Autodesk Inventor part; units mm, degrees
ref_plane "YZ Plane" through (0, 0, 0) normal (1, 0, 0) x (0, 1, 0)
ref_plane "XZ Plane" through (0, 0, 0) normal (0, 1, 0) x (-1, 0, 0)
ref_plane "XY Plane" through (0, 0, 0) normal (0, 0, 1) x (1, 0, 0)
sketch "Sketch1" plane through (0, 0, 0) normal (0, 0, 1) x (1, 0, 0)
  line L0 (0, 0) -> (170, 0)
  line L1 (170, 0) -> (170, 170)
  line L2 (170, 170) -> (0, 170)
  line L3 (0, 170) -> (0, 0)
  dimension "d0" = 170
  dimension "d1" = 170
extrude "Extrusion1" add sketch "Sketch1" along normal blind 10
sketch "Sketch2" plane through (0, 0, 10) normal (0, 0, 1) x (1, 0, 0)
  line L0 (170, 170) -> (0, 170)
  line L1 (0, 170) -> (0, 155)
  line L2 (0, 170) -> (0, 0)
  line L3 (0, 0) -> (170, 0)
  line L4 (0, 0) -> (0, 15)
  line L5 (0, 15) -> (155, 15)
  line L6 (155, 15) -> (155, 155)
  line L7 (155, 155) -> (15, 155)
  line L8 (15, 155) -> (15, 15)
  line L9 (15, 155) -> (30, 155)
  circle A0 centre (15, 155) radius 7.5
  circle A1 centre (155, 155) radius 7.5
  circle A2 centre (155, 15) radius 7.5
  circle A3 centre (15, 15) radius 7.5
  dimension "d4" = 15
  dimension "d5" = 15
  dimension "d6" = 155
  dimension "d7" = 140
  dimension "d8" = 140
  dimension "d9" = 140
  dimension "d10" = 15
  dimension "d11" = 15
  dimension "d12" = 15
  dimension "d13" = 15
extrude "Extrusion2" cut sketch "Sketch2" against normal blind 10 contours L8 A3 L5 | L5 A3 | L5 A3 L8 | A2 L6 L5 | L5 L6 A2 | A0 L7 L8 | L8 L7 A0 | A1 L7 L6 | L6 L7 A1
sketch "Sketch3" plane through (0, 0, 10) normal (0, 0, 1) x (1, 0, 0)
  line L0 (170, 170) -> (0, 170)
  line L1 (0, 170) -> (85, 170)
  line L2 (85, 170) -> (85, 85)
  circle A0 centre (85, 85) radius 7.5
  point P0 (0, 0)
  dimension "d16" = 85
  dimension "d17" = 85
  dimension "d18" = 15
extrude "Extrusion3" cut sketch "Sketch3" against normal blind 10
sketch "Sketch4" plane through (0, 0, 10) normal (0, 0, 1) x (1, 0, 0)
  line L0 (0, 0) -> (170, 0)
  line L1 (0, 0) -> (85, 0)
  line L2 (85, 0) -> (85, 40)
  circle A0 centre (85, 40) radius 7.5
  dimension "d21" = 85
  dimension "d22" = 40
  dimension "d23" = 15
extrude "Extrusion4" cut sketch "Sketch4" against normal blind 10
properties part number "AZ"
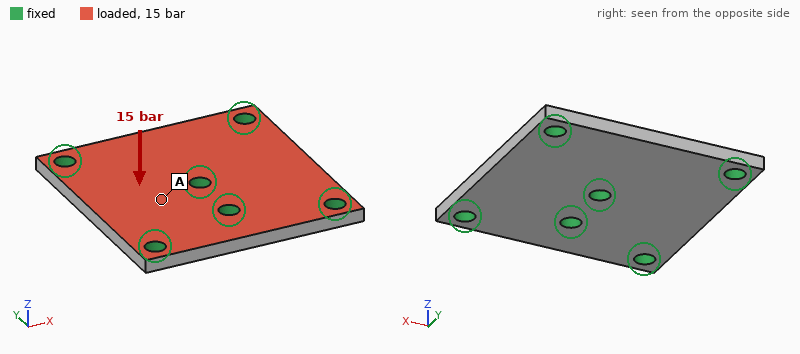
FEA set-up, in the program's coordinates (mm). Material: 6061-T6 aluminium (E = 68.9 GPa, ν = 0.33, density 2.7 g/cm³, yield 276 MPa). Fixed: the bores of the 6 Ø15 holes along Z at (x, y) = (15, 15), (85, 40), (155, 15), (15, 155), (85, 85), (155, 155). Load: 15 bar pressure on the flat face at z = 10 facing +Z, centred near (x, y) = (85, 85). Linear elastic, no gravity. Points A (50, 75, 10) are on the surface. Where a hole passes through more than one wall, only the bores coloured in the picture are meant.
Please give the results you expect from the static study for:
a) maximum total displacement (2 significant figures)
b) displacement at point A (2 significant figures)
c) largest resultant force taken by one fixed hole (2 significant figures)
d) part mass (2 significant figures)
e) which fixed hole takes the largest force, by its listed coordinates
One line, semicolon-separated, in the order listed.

0.18 mm; 0.065 mm; 11 kN; 750 g; (85, 85)
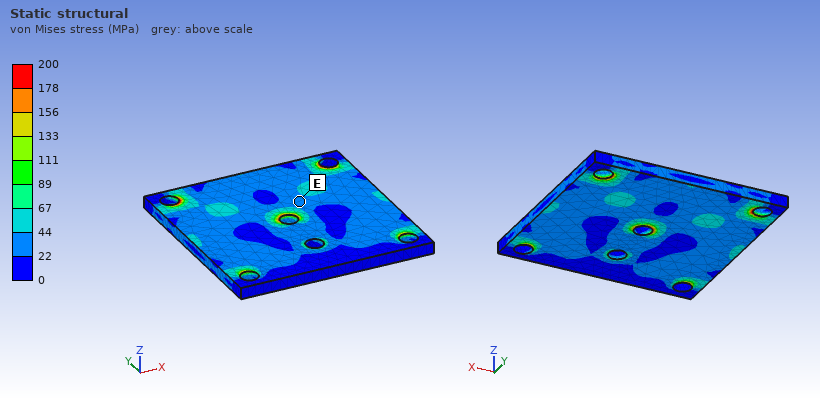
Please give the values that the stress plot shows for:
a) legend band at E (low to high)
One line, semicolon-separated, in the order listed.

22 to 44 MPa
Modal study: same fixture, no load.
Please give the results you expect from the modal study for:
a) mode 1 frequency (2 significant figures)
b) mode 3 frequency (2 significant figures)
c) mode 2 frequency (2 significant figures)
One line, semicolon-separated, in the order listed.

3400 Hz; 3700 Hz; 3600 Hz
